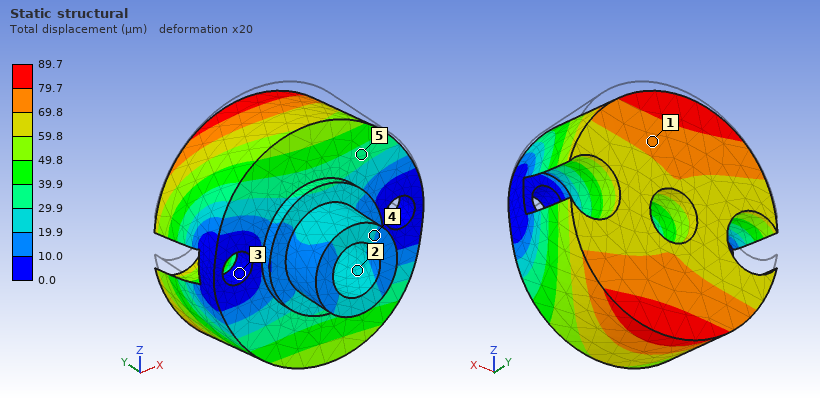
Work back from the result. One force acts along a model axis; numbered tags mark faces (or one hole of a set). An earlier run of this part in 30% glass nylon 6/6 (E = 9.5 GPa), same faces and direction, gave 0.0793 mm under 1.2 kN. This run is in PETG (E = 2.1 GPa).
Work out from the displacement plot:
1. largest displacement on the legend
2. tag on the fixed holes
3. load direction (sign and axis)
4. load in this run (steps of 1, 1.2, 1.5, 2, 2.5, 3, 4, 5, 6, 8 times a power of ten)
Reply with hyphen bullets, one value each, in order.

- 89.7 µm
- 3
- -Z
- 300 N
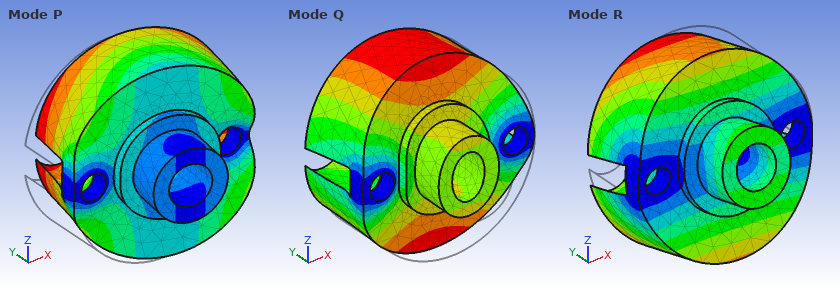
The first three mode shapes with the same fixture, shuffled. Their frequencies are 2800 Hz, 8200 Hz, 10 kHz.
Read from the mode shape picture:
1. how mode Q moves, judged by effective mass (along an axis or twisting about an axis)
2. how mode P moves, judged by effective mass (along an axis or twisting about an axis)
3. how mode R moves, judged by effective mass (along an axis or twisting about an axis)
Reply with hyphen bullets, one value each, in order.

- along Y
- along X
- along Z
